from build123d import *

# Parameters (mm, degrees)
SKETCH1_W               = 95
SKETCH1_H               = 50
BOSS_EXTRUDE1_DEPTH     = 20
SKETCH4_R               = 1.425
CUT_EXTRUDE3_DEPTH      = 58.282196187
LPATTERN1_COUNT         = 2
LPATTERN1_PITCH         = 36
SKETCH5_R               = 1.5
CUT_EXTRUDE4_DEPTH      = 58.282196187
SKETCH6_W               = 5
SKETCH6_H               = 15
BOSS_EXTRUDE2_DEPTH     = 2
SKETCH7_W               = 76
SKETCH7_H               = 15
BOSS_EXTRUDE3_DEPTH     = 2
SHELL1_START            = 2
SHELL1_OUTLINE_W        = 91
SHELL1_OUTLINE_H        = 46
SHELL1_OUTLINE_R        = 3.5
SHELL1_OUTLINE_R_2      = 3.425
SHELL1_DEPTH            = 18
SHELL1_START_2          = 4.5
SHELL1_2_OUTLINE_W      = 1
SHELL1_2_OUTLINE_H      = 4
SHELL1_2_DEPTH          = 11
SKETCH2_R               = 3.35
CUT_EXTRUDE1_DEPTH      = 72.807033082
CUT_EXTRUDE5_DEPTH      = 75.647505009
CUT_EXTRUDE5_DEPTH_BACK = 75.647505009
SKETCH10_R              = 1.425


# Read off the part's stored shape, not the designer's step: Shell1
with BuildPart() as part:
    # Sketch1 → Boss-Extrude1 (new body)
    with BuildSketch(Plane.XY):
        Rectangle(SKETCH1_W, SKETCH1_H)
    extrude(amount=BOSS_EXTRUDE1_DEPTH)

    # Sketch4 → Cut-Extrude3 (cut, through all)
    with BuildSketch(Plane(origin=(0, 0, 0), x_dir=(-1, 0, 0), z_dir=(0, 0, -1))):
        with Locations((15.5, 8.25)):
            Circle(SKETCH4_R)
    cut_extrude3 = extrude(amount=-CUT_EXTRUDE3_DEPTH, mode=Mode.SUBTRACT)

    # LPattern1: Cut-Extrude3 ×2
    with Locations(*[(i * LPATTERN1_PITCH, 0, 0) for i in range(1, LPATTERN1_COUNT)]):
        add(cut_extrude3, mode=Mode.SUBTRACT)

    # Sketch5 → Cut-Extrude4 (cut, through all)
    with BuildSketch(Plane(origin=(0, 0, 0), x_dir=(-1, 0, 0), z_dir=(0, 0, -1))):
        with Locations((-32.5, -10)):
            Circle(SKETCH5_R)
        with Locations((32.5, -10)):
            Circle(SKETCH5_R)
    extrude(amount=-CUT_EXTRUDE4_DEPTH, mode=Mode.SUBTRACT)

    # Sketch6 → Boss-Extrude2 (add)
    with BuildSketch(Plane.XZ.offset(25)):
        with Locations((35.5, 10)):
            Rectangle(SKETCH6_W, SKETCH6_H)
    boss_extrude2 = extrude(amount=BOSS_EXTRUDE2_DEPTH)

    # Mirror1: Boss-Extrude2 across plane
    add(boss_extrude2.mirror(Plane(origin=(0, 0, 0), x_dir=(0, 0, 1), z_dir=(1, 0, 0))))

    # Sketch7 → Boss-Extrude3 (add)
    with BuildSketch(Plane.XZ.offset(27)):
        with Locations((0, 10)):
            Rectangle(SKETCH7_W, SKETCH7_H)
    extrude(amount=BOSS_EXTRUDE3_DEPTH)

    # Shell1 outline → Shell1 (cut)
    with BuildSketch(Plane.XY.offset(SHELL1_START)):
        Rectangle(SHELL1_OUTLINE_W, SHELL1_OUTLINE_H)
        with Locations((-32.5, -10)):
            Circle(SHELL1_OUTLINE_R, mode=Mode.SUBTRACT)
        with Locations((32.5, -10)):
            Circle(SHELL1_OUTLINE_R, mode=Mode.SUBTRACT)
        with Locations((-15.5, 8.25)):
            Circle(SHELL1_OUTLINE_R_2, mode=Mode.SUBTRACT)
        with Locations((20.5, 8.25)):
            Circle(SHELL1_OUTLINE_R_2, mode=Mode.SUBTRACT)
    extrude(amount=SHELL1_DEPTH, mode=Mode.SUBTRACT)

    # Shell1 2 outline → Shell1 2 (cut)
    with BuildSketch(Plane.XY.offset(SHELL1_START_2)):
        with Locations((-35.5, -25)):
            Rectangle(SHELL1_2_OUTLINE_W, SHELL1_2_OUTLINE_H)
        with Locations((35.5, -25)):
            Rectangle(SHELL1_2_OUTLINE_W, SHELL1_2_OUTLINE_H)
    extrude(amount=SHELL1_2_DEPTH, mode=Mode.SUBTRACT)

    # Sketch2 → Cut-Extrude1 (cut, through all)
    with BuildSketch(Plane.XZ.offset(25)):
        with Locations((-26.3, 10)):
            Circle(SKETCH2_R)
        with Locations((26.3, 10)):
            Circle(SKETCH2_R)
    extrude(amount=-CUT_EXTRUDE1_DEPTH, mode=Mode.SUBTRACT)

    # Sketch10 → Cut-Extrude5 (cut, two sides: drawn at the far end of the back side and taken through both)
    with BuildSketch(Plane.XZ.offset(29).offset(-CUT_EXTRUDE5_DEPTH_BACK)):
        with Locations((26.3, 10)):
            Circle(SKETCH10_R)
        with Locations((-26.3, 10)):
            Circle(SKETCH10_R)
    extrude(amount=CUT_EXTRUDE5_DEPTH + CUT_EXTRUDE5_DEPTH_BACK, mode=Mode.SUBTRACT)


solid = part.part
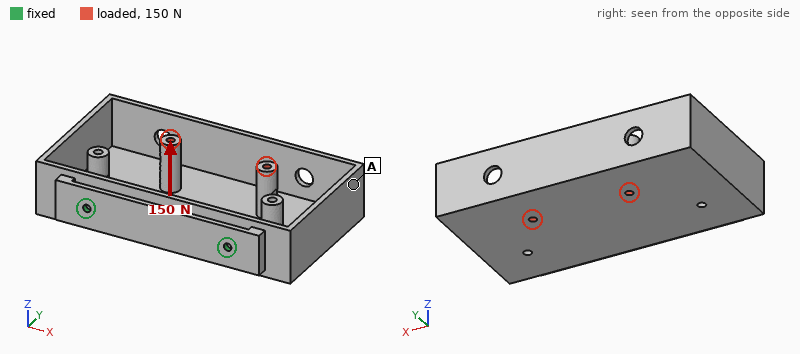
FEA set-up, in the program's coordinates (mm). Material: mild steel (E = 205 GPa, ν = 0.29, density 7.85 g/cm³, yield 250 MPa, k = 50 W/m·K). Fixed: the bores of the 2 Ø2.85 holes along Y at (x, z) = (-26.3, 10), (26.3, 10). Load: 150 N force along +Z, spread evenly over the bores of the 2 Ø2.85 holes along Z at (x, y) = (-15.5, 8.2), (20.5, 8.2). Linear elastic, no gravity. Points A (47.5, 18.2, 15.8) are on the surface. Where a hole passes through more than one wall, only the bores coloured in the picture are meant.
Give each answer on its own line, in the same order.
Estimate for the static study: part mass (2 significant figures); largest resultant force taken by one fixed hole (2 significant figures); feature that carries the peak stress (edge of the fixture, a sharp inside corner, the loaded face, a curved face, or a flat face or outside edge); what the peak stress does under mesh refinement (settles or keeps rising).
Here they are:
190 g
140 N
edge of the fixture
keeps rising
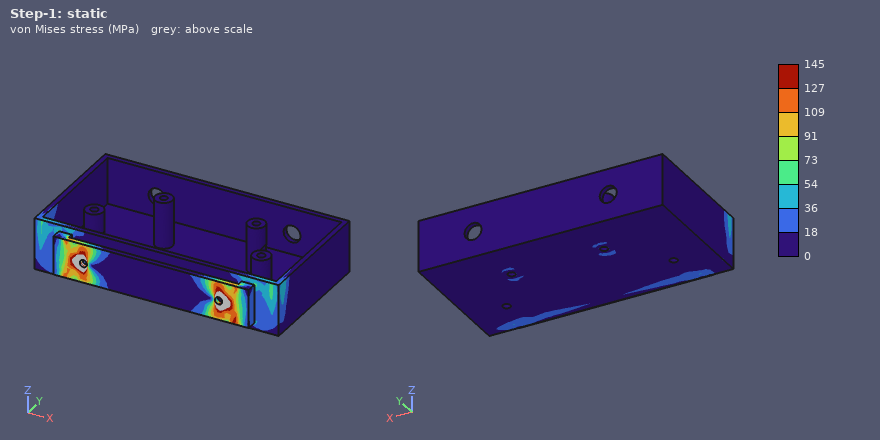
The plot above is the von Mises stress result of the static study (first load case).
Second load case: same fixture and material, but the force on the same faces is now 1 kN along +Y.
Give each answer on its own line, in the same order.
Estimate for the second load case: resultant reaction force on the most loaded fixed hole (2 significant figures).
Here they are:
820 N
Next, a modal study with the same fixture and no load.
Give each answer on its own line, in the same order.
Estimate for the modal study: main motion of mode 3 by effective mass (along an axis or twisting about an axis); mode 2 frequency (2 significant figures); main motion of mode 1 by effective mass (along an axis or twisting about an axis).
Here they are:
along X
720 Hz
along Z
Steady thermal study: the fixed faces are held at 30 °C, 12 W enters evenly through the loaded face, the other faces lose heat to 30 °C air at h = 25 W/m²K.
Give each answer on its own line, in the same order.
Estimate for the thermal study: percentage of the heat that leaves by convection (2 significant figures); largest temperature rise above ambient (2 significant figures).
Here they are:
83 %
66 K
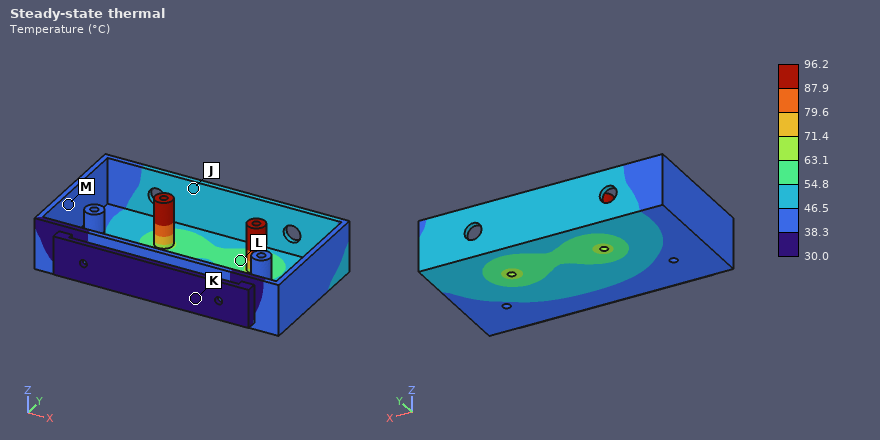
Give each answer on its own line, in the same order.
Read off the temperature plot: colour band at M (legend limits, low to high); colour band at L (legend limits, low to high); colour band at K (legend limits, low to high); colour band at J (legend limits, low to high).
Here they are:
38.3 to 46.5 °C
54.8 to 63.1 °C
30.0 to 38.3 °C
46.5 to 54.8 °C
